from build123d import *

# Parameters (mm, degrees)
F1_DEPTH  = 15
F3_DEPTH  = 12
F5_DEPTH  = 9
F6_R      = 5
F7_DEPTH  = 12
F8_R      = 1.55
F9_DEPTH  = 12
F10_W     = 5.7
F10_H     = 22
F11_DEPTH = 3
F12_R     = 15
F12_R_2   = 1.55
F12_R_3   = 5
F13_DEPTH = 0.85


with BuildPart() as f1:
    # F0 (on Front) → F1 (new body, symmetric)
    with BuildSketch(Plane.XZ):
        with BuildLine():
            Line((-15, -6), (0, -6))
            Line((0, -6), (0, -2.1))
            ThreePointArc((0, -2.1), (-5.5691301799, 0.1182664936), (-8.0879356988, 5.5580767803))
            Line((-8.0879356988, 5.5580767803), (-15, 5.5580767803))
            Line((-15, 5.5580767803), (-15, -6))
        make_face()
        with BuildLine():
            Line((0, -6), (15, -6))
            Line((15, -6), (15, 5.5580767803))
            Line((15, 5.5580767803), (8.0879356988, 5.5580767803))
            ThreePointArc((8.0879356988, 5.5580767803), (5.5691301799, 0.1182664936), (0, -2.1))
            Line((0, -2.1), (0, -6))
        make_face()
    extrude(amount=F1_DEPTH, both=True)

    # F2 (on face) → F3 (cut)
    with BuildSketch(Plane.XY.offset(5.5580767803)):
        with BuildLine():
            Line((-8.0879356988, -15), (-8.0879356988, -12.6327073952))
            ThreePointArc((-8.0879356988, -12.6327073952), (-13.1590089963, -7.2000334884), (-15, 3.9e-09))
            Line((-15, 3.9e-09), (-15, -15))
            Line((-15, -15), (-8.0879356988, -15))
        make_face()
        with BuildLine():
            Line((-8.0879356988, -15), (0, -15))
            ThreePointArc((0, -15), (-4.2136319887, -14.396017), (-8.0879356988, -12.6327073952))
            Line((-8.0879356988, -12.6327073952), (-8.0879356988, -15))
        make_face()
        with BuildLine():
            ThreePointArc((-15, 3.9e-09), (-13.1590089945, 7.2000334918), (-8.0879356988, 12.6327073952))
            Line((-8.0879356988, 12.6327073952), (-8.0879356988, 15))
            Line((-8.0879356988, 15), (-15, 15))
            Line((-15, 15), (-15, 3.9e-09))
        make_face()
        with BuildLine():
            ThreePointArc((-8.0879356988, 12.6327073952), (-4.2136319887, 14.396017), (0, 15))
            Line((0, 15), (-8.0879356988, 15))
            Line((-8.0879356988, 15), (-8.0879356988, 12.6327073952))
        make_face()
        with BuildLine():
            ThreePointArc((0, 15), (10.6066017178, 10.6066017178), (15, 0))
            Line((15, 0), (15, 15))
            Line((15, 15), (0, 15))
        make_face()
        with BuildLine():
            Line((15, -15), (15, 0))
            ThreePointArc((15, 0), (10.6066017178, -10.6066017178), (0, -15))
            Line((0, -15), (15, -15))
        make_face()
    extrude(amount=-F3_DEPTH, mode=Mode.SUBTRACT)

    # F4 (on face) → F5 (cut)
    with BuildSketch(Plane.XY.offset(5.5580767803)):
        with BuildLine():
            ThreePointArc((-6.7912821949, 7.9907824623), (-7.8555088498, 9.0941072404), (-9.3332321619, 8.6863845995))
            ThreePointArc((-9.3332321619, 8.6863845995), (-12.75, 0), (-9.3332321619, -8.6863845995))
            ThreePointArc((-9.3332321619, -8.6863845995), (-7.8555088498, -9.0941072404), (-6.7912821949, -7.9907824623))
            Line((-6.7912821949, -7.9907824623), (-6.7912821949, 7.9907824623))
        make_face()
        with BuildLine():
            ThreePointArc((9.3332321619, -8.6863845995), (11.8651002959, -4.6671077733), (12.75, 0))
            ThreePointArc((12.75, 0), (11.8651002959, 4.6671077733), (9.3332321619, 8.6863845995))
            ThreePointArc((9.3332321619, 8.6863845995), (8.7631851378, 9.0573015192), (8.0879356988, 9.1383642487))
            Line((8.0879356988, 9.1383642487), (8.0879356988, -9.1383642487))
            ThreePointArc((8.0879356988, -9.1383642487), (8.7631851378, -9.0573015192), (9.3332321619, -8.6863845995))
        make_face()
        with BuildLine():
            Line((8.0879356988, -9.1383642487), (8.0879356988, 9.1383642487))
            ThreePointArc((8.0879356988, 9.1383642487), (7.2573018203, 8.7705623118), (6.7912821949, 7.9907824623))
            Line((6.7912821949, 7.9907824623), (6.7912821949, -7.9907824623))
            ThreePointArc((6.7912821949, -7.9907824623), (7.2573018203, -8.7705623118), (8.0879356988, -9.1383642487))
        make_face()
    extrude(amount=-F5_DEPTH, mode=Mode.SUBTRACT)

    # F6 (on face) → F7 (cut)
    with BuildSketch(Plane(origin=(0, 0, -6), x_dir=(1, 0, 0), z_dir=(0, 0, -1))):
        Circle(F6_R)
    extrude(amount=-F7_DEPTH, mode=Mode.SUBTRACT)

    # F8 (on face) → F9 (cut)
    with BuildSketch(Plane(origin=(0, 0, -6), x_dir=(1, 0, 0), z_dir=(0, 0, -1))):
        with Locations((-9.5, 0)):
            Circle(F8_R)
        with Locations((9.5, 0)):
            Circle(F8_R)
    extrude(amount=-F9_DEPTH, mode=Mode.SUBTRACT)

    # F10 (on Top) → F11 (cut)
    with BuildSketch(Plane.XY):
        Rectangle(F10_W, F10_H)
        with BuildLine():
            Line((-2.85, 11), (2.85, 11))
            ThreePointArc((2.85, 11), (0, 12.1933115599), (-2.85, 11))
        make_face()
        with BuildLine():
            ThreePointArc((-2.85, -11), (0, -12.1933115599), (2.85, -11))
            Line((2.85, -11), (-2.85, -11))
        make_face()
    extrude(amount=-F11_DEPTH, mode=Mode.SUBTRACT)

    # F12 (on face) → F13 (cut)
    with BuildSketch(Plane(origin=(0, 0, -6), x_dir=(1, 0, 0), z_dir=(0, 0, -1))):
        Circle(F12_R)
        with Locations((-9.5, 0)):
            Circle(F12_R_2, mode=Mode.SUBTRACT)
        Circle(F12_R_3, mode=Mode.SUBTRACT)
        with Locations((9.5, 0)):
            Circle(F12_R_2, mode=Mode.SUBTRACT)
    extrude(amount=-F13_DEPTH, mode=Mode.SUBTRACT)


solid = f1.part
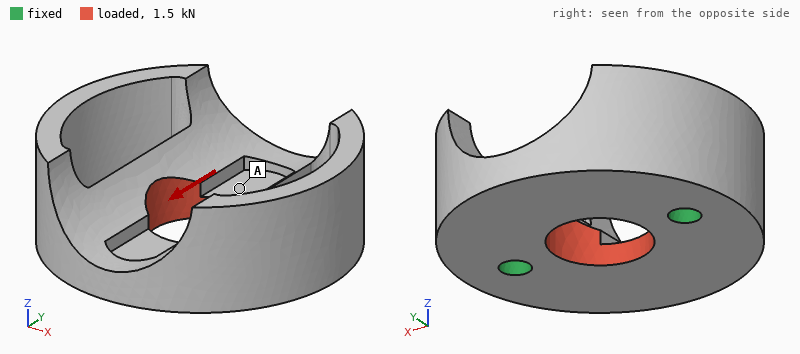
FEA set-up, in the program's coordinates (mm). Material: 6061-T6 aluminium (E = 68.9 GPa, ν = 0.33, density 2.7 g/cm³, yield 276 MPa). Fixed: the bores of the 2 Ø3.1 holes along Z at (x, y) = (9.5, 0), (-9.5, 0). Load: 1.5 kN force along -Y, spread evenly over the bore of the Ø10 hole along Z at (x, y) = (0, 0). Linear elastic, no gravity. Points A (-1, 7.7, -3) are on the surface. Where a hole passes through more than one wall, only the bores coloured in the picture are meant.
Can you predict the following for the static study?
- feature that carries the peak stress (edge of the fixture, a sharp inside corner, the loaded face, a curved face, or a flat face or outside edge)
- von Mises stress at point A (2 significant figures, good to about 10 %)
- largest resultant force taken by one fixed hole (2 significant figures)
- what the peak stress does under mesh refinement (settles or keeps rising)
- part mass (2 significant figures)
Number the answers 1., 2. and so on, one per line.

1. edge of the fixture
2. 13 MPa
3. 750 N
4. keeps rising
5. 8.0 g
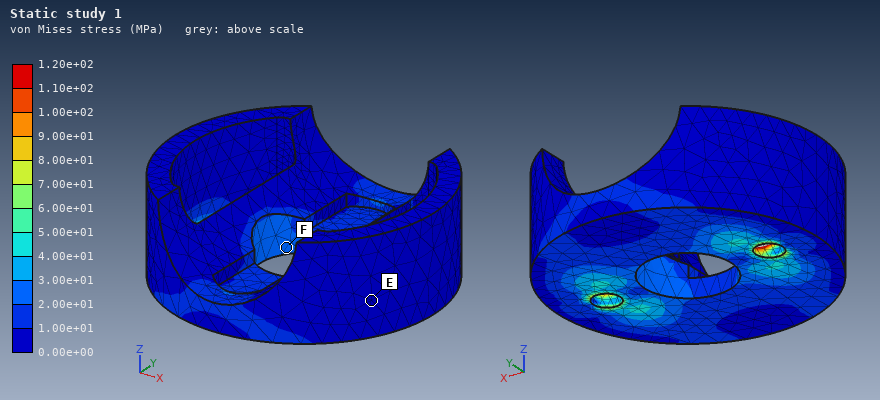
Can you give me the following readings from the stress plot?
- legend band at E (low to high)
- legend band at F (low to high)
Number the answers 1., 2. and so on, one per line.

1. 0.00e+00 to 1.00e+01 MPa
2. 2.00e+01 to 3.00e+01 MPa
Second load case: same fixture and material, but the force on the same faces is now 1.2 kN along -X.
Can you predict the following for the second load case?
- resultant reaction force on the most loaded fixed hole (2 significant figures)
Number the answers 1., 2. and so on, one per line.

1. 600 N
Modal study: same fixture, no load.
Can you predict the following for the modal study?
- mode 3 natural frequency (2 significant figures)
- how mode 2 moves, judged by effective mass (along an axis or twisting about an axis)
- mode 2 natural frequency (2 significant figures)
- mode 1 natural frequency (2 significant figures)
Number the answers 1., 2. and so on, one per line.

1. 15 kHz
2. along Z
3. 12 kHz
4. 6200 Hz
